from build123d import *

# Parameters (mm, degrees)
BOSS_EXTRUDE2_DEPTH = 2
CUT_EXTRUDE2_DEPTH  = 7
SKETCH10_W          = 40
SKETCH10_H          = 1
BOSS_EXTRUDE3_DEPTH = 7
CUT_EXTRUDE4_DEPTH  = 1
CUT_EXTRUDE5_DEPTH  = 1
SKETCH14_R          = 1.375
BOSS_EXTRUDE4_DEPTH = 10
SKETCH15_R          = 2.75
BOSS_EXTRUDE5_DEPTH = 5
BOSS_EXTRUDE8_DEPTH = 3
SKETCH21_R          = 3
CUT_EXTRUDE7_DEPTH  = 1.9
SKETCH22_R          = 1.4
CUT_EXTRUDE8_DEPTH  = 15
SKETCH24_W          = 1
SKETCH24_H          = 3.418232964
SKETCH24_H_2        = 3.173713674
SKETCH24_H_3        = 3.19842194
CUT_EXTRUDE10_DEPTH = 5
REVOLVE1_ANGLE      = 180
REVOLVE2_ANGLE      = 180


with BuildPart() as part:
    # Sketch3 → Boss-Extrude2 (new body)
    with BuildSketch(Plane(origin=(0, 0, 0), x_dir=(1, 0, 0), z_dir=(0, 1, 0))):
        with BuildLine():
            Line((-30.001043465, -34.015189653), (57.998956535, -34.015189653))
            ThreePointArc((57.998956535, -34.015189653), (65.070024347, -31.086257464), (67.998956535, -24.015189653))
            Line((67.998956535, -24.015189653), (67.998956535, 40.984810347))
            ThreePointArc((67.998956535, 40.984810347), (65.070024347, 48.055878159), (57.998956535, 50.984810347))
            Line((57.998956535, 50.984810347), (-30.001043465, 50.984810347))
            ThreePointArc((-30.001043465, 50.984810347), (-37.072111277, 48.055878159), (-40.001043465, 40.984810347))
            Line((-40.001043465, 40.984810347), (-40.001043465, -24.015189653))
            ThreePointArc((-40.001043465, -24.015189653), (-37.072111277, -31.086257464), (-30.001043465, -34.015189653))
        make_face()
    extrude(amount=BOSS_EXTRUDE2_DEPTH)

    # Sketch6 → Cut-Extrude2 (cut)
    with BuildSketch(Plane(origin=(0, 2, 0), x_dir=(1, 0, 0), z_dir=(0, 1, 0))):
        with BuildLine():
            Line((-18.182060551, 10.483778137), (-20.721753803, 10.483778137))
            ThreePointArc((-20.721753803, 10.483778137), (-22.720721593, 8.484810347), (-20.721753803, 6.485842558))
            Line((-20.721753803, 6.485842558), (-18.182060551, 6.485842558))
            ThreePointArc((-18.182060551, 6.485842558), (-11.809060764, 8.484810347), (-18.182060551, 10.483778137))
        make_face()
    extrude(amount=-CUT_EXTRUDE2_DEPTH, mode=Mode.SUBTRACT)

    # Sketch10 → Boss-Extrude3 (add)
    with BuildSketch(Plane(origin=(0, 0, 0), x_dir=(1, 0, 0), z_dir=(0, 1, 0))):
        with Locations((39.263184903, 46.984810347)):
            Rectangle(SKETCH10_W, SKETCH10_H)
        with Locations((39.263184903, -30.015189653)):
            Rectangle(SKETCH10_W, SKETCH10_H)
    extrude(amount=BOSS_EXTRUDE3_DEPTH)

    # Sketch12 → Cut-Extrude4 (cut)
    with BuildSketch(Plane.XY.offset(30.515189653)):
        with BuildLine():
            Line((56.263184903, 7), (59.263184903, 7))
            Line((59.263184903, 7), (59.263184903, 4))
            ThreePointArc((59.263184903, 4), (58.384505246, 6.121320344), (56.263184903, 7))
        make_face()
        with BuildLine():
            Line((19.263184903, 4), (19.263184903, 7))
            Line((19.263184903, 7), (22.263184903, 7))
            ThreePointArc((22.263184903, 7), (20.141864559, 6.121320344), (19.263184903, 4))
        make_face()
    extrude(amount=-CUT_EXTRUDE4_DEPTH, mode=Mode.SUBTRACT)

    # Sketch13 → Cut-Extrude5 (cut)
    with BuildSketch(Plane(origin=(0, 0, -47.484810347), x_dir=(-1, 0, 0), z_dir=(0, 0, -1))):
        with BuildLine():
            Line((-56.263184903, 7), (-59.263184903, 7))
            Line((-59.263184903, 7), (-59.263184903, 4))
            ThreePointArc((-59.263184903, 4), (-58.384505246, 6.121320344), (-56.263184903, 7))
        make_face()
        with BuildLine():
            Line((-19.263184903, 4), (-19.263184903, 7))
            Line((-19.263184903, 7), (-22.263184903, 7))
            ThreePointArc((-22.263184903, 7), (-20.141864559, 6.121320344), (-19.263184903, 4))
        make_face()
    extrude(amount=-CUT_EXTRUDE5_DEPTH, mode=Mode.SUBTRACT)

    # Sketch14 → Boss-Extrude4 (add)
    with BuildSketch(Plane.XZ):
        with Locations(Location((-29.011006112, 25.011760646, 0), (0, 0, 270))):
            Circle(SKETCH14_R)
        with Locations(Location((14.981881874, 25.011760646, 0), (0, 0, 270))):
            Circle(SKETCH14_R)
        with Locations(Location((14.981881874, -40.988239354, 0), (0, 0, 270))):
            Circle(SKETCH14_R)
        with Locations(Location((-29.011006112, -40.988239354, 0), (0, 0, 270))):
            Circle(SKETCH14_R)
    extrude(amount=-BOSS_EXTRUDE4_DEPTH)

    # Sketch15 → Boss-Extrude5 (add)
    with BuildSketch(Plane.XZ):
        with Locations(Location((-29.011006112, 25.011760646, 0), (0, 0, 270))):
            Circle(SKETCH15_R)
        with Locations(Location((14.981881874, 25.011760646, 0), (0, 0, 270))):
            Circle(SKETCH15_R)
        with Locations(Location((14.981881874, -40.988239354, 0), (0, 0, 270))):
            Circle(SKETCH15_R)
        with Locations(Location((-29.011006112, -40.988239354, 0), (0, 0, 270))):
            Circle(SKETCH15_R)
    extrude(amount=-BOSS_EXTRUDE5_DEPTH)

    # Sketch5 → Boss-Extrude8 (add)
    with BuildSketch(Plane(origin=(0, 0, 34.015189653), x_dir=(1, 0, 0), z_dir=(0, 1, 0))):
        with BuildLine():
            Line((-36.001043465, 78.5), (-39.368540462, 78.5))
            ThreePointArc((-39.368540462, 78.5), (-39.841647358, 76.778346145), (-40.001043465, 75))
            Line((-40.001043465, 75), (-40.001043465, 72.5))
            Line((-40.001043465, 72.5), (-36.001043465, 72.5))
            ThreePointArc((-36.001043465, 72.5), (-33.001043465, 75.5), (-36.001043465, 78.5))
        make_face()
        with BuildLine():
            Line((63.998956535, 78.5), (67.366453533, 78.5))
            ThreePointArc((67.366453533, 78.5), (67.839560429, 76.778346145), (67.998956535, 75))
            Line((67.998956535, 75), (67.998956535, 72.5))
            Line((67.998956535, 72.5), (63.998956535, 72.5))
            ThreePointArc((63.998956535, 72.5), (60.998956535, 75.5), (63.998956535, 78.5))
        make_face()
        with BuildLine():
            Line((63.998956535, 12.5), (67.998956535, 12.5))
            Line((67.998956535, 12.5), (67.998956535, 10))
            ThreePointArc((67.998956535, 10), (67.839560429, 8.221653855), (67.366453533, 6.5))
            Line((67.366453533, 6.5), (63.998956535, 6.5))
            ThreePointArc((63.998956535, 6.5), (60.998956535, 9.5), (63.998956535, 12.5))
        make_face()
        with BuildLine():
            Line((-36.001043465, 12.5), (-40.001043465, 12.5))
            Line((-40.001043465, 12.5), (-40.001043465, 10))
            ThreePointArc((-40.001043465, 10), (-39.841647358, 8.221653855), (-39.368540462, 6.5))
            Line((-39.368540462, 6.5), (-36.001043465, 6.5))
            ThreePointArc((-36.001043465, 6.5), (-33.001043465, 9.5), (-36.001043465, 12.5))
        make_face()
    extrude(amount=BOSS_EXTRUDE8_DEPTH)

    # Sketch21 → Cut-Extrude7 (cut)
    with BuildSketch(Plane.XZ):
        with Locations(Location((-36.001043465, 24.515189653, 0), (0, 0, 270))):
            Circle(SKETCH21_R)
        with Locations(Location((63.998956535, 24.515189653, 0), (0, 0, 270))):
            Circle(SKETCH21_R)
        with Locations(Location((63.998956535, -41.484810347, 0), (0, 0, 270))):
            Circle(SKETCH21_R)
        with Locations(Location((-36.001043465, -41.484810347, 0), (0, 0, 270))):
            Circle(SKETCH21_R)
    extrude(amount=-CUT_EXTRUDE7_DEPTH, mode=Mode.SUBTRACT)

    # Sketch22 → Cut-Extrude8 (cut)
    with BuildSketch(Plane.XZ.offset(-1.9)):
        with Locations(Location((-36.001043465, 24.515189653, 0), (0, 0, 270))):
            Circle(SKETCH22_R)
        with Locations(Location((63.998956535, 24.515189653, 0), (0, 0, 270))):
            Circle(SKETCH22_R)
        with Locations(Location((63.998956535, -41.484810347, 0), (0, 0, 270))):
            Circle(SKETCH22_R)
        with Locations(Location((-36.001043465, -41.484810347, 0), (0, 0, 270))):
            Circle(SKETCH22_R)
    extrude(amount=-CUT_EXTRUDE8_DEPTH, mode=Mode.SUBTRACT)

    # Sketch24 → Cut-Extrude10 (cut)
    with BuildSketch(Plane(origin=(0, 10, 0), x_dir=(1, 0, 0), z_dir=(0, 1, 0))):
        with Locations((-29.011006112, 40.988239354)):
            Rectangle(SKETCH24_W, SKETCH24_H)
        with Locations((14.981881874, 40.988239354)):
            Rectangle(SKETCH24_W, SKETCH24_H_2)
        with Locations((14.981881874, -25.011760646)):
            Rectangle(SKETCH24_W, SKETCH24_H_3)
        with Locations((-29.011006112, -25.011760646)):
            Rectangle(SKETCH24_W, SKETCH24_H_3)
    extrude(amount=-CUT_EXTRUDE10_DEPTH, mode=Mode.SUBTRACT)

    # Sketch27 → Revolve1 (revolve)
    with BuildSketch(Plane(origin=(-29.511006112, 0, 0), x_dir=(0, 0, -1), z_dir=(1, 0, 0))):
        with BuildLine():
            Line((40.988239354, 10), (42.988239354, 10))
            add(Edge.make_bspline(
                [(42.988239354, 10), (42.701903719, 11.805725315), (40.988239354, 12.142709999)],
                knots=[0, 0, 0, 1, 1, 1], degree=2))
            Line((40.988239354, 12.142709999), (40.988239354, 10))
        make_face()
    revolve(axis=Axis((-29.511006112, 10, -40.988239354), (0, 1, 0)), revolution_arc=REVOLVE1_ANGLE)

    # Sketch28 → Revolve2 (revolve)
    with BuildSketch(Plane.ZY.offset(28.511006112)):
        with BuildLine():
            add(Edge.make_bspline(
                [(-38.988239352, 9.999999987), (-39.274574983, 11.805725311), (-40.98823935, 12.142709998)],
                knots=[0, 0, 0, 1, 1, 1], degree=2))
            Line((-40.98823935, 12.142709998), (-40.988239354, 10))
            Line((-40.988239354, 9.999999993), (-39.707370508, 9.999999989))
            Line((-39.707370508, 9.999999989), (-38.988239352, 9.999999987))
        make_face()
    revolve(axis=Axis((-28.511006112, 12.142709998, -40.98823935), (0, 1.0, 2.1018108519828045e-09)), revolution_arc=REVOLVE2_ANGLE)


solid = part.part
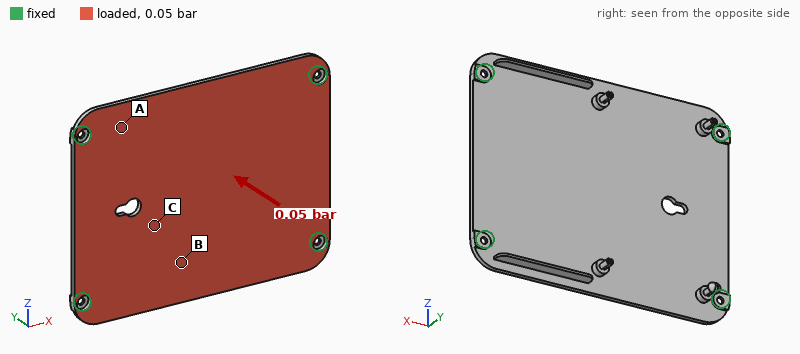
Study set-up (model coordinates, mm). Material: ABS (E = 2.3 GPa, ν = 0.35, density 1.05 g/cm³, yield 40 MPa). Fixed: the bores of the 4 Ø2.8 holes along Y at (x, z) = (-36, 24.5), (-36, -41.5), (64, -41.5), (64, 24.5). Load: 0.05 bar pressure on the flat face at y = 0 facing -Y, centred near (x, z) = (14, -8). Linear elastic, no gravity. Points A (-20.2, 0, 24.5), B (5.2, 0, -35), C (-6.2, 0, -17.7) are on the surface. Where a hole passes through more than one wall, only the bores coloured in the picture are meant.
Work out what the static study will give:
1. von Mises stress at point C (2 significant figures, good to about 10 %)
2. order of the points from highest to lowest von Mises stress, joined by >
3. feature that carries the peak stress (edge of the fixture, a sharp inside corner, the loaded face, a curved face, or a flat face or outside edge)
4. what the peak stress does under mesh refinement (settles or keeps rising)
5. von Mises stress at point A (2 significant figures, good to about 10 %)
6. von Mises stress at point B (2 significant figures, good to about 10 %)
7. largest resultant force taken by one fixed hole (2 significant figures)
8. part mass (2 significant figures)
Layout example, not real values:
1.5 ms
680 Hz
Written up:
3.0 MPa
B > C > A
a sharp inside corner
keeps rising
1.4 MPa
4.4 MPa
43 N
20 g
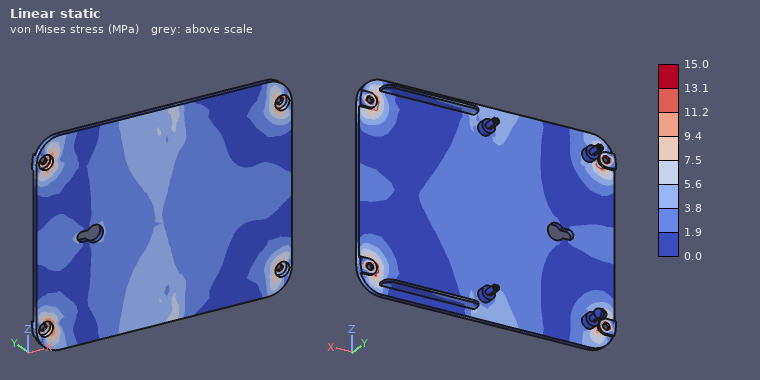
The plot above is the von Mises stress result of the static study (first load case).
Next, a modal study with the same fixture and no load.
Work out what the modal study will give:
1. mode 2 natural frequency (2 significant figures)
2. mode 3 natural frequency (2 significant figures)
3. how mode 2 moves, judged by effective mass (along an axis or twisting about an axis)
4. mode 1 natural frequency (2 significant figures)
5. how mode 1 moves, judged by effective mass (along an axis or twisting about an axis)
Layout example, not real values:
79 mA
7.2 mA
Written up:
350 Hz
550 Hz
twisting about X
240 Hz
along Y
